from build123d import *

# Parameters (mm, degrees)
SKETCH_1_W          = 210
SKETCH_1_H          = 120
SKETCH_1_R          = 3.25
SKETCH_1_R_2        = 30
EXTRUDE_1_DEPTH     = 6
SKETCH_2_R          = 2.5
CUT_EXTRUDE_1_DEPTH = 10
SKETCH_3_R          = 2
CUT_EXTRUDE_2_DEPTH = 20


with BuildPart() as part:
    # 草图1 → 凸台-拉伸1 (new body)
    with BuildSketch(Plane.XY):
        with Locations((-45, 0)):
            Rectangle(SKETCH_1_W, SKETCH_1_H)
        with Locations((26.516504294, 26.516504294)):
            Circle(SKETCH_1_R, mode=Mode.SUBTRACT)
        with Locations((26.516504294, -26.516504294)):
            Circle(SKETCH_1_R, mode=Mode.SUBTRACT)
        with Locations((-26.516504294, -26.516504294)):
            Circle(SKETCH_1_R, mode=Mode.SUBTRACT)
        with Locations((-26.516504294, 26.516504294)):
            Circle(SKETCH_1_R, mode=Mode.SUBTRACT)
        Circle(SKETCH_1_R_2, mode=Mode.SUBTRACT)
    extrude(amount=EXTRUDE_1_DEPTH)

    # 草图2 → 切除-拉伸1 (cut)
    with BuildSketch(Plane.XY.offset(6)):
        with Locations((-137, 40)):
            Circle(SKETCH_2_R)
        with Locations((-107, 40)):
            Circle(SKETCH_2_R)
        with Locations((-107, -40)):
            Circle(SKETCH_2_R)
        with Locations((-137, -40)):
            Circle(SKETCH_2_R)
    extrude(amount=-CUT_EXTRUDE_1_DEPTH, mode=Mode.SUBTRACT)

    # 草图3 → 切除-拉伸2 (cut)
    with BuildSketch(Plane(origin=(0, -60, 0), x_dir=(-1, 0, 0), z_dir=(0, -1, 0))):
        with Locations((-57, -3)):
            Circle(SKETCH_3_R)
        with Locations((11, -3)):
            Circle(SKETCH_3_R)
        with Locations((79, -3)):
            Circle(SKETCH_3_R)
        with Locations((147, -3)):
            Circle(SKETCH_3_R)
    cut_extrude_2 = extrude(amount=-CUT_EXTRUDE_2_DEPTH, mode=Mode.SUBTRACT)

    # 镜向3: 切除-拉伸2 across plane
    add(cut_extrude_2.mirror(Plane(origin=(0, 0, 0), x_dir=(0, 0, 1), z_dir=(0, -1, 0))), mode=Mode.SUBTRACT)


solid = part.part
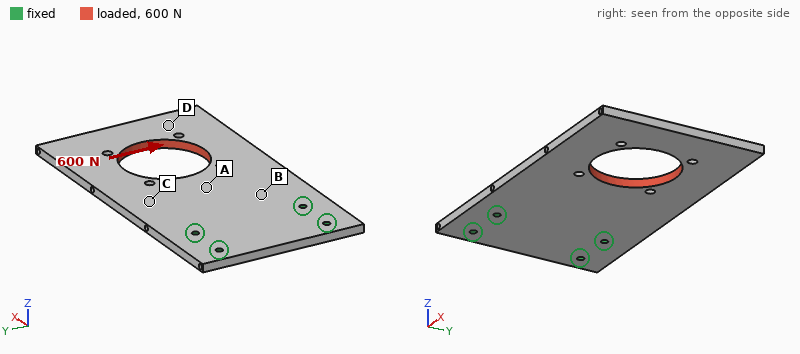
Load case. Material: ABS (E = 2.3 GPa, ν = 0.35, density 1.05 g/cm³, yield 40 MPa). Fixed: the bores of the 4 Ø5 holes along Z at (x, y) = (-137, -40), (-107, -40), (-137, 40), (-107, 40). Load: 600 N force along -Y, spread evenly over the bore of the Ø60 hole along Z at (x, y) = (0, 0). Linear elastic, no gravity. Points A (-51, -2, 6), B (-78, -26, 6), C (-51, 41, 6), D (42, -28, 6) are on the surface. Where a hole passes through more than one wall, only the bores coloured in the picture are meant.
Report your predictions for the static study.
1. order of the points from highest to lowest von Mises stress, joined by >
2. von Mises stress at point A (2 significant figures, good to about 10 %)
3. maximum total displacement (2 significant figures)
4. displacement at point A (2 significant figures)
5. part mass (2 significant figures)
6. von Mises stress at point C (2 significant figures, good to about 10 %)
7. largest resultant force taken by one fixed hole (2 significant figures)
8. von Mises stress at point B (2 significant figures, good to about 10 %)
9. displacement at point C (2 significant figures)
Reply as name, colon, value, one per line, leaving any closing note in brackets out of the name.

order of the points from highest to lowest von Mises stress, joined by >: A > B > C > D
von Mises stress at point A: 3.4 MPa
maximum total displacement: 0.66 mm
displacement at point A: 0.15 mm
part mass: 140 g
von Mises stress at point C: 1.4 MPa
largest resultant force taken by one fixed hole: 650 N
von Mises stress at point B: 2.4 MPa
displacement at point C: 0.16 mm
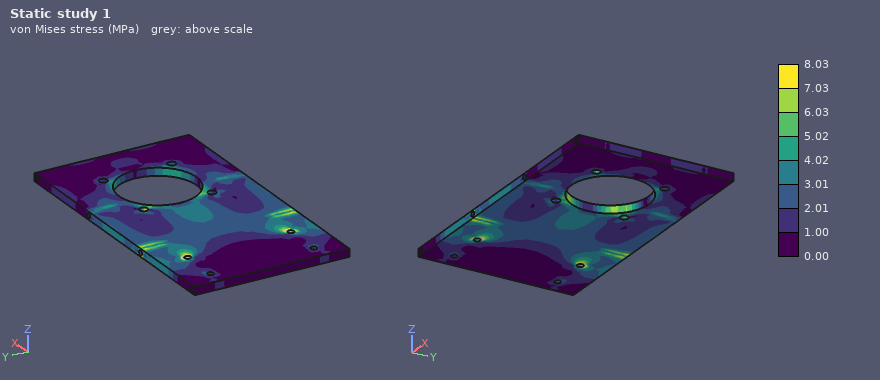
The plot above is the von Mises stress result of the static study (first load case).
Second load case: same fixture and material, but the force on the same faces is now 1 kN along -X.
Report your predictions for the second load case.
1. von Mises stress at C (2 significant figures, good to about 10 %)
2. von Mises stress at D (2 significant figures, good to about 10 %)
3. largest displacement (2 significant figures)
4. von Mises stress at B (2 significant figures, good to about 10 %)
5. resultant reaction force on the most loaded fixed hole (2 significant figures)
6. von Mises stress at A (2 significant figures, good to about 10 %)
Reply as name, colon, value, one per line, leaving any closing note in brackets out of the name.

von Mises stress at C: 1.7 MPa
von Mises stress at D: 1.2 MPa
largest displacement: 0.17 mm
von Mises stress at B: 1.3 MPa
resultant reaction force on the most loaded fixed hole: 360 N
von Mises stress at A: 1.0 MPa
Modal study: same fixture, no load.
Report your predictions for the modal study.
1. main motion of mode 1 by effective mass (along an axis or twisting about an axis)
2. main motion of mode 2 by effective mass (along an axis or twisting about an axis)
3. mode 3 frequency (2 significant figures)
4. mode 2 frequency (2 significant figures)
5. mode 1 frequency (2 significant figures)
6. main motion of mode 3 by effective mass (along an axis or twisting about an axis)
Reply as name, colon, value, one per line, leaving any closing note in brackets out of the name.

main motion of mode 1 by effective mass: along Z
main motion of mode 2 by effective mass: twisting about X
mode 3 frequency: 280 Hz
mode 2 frequency: 150 Hz
mode 1 frequency: 53 Hz
main motion of mode 3 by effective mass: along Z
